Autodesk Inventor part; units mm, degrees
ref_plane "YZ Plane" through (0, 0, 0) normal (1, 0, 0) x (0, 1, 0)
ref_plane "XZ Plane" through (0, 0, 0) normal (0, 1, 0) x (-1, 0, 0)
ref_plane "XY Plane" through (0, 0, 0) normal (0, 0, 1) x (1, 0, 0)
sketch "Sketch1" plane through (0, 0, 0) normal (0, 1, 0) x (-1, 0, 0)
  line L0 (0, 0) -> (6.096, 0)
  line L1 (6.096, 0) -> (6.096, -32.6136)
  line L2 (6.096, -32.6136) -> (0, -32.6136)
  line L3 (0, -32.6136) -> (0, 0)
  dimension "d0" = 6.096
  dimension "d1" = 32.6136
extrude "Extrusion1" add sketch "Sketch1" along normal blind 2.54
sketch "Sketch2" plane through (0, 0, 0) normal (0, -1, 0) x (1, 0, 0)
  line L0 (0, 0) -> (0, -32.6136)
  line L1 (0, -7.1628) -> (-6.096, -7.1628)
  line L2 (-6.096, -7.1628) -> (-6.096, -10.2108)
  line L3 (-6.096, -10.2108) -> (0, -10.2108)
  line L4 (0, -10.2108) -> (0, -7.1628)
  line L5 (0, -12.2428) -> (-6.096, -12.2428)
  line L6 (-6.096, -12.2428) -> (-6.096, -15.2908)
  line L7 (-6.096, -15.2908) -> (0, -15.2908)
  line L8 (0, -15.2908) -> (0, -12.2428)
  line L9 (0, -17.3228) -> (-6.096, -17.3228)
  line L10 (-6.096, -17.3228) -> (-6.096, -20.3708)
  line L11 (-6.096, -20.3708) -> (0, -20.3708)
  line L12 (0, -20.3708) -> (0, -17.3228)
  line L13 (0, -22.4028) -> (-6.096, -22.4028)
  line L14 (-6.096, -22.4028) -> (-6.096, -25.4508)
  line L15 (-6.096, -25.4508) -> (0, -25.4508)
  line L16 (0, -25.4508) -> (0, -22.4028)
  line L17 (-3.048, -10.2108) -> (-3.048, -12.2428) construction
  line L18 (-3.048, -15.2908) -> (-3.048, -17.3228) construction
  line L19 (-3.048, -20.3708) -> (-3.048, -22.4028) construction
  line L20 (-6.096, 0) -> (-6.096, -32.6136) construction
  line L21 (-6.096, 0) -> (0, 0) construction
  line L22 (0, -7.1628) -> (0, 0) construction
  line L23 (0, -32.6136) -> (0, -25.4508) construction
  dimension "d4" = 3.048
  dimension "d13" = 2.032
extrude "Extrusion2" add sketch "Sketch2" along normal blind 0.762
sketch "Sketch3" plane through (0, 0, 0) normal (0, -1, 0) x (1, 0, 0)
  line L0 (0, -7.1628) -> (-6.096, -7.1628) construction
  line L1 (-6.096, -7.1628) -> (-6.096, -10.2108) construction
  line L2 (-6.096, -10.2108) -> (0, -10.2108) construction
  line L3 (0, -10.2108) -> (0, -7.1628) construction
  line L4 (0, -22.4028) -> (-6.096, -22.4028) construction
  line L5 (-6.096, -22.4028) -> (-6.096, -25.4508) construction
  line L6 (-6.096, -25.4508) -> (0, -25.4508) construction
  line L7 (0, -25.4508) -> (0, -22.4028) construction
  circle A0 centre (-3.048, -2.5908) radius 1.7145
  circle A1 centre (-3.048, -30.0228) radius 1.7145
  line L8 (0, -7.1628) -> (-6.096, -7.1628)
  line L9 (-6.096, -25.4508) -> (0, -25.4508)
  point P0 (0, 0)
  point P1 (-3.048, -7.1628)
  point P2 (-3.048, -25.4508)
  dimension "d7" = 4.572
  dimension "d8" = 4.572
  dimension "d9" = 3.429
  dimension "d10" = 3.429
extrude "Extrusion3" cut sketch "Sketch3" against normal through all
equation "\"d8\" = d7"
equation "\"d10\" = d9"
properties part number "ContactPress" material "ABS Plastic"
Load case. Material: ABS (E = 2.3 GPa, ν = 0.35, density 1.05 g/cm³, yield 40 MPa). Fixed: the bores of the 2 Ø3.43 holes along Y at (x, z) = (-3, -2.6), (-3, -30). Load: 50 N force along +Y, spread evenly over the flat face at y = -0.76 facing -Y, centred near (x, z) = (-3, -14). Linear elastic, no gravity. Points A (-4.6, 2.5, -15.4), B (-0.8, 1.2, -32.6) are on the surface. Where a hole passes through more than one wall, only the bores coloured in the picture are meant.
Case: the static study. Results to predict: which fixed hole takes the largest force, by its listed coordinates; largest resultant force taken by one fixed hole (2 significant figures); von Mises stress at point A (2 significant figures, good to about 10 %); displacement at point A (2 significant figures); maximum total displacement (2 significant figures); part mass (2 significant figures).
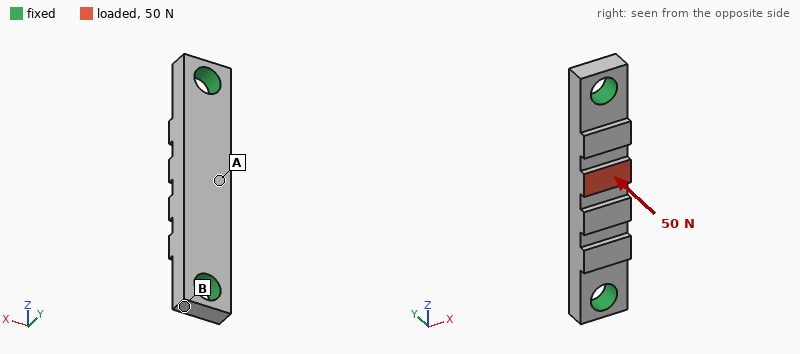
(-3, -2.6)
33 N
16 MPa
0.18 mm
0.19 mm
0.54 g
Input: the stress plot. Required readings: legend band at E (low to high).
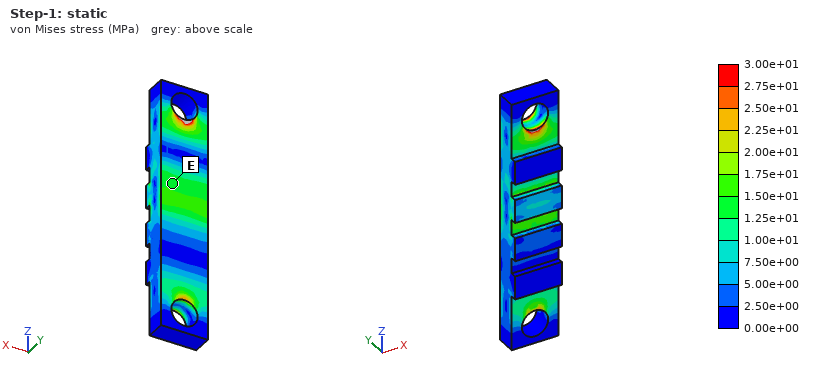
1.25e+01 to 1.50e+01 MPa
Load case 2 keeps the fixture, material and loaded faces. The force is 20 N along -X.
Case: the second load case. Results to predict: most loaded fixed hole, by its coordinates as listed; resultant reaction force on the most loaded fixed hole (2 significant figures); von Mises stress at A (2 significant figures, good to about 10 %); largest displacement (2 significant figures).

(-3, -2.6)
13 N
2.3 MPa
50 µm
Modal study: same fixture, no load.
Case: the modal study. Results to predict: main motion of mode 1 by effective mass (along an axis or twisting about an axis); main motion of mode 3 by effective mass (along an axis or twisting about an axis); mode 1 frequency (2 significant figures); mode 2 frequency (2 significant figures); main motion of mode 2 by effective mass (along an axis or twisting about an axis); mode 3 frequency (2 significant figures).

along Y
twisting about Z
5600 Hz
9300 Hz
along X
12 kHz
